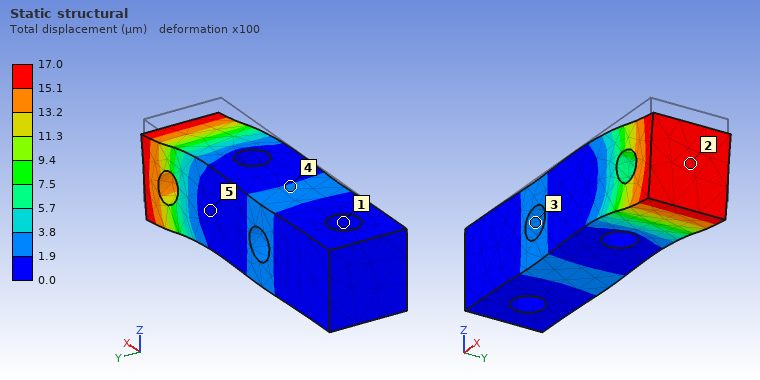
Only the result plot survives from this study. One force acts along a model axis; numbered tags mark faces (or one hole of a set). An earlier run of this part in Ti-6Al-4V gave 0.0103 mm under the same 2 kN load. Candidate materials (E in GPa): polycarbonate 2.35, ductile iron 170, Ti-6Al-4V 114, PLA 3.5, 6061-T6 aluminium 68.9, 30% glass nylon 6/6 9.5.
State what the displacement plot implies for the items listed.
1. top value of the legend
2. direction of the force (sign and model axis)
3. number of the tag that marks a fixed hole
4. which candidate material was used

17.0 µm
-Z
1
6061-T6 aluminium
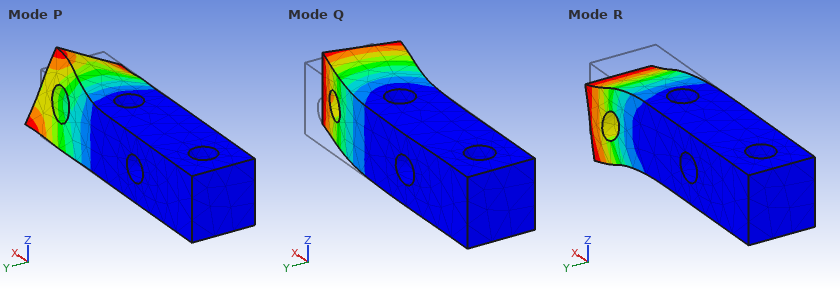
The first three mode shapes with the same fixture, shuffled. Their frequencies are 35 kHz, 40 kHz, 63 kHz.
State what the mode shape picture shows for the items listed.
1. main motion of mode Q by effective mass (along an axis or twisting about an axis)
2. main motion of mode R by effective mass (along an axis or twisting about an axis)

along Y
along Z
